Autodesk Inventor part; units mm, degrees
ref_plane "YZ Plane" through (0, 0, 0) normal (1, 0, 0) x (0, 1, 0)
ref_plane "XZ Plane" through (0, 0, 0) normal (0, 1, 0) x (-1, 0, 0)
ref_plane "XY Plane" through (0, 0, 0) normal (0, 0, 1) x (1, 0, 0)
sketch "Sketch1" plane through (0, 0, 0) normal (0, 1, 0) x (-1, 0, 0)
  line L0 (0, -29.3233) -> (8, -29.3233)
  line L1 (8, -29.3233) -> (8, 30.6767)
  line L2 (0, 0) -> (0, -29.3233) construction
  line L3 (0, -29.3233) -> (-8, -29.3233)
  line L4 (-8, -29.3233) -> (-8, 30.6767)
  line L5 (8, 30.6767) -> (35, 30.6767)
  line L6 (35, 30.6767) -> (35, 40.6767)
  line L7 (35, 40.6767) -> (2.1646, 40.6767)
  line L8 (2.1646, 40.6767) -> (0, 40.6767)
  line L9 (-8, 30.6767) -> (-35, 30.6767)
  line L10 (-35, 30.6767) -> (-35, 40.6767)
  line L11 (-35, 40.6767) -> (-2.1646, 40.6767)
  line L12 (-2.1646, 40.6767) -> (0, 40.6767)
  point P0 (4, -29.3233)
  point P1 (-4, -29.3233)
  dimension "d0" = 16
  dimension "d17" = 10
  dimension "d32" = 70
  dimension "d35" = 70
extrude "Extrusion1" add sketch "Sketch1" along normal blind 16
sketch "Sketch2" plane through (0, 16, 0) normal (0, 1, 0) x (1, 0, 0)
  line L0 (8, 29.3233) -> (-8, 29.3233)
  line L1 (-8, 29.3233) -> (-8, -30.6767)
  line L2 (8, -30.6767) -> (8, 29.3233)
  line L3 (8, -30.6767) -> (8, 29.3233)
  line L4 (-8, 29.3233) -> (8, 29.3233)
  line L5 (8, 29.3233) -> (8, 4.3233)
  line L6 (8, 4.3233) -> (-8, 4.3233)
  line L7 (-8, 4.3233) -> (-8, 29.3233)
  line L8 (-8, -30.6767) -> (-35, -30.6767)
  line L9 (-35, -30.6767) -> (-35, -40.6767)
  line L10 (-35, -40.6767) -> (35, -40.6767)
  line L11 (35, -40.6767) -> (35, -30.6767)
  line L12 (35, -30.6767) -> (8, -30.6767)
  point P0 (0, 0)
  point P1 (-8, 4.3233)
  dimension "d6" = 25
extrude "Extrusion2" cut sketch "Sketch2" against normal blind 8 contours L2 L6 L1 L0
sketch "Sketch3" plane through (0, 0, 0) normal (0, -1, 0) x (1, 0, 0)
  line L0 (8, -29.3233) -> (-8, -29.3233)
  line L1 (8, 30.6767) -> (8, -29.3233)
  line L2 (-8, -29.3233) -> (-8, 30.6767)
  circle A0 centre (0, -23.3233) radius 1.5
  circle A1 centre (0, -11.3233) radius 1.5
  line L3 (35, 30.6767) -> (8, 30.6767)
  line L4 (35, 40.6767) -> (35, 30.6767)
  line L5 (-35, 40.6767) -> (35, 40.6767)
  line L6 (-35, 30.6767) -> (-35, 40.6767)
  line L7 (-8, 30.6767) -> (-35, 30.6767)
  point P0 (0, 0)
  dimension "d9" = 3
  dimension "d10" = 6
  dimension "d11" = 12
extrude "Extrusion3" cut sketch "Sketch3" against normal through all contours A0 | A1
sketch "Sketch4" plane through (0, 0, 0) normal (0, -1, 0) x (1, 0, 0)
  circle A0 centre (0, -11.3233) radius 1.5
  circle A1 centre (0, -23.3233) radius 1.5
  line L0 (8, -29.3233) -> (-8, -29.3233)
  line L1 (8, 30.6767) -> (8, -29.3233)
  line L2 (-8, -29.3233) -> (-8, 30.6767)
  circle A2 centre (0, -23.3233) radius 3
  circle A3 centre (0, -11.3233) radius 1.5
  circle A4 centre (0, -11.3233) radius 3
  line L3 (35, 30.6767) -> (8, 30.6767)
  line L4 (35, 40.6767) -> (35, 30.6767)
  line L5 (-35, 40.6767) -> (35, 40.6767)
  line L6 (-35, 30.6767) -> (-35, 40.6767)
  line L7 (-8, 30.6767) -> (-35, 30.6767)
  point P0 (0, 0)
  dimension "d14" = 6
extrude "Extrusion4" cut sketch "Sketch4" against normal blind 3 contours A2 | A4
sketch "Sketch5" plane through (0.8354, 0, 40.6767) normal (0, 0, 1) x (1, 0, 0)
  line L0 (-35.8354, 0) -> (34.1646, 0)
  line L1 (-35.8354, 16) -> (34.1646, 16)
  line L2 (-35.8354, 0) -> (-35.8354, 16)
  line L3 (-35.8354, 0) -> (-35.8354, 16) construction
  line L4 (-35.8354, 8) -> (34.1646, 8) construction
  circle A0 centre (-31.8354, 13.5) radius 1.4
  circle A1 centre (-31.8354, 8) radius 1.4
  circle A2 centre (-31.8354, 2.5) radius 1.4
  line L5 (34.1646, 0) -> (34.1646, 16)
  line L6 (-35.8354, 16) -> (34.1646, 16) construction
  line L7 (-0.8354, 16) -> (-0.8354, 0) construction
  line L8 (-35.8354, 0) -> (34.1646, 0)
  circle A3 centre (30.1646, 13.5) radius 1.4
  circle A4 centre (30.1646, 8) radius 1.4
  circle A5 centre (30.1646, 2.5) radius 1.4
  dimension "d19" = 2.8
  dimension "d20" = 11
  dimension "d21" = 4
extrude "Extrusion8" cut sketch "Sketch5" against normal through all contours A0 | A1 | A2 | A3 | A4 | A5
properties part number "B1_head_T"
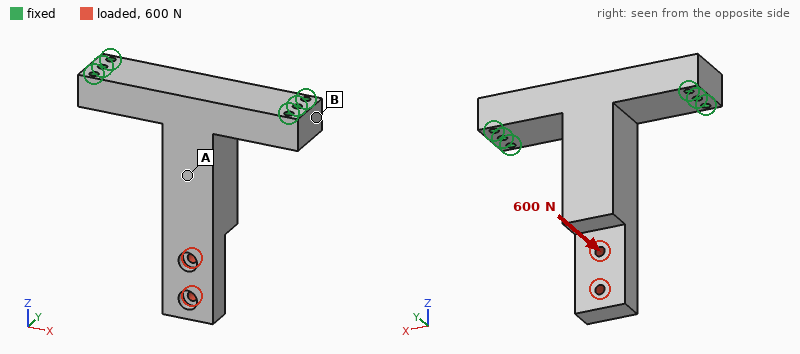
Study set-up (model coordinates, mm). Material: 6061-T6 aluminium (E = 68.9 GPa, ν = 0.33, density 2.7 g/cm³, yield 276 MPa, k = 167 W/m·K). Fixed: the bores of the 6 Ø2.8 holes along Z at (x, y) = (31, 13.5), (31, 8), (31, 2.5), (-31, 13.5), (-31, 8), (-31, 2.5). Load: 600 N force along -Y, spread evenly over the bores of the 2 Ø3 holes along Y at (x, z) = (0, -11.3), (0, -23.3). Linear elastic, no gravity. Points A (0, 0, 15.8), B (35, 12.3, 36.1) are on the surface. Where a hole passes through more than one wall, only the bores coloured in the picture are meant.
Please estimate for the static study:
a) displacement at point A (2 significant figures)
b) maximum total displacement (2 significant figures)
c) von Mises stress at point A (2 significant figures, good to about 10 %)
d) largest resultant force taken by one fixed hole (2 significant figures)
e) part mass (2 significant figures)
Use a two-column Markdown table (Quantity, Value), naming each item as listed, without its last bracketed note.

| Quantity | Value |
|---|---|
| displacement at point A | 0.11 mm |
| maximum total displacement | 0.42 mm |
| von Mises stress at point A | 29 MPa |
| largest resultant force taken by one fixed hole | 970 N |
| part mass | 61 g |
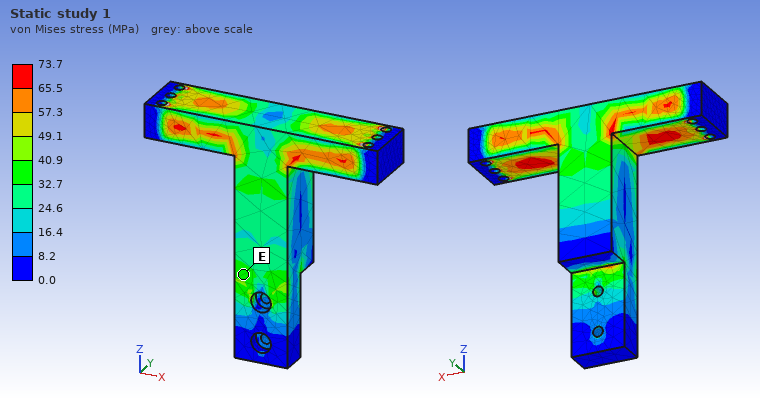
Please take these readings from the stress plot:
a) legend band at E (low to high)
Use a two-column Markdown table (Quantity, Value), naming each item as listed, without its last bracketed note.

| Quantity | Value |
|---|---|
| legend band at E | 32.7 to 40.9 MPa |
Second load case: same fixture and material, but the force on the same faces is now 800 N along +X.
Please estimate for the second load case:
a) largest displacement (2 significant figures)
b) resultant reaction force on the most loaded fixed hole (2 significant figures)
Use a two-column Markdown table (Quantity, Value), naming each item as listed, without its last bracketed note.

| Quantity | Value |
|---|---|
| largest displacement | 0.22 mm |
| resultant reaction force on the most loaded fixed hole | 380 N |
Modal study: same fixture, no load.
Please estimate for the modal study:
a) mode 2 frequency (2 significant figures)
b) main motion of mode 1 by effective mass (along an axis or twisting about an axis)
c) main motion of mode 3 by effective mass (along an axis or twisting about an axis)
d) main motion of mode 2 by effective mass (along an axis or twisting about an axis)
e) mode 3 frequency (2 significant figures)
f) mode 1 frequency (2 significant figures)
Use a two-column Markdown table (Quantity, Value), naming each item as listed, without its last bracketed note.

| Quantity | Value |
|---|---|
| mode 2 frequency | 3300 Hz |
| main motion of mode 1 by effective mass | along Y |
| main motion of mode 3 by effective mass | along Z |
| main motion of mode 2 by effective mass | along X |
| mode 3 frequency | 7000 Hz |
| mode 1 frequency | 1900 Hz |
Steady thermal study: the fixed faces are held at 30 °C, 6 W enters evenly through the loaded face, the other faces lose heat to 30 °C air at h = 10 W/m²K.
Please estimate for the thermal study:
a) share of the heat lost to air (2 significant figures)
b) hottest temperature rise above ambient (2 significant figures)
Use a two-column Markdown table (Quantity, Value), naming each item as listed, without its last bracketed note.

| Quantity | Value |
|---|---|
| share of the heat lost to air | 5.4 % |
| hottest temperature rise above ambient | 13 K |
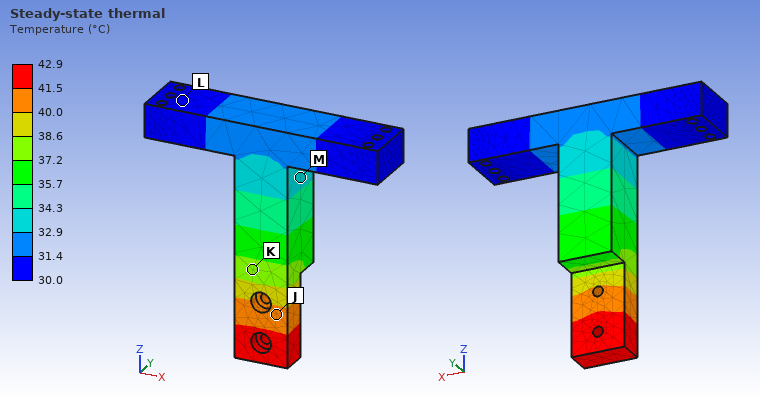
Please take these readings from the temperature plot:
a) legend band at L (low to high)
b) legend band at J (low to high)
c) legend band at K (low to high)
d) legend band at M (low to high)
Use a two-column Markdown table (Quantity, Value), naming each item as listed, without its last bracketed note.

| Quantity | Value |
|---|---|
| legend band at L | 30.0 to 31.4 °C |
| legend band at J | 40.0 to 41.5 °C |
| legend band at K | 37.2 to 38.6 °C |
| legend band at M | 32.9 to 34.3 °C |
